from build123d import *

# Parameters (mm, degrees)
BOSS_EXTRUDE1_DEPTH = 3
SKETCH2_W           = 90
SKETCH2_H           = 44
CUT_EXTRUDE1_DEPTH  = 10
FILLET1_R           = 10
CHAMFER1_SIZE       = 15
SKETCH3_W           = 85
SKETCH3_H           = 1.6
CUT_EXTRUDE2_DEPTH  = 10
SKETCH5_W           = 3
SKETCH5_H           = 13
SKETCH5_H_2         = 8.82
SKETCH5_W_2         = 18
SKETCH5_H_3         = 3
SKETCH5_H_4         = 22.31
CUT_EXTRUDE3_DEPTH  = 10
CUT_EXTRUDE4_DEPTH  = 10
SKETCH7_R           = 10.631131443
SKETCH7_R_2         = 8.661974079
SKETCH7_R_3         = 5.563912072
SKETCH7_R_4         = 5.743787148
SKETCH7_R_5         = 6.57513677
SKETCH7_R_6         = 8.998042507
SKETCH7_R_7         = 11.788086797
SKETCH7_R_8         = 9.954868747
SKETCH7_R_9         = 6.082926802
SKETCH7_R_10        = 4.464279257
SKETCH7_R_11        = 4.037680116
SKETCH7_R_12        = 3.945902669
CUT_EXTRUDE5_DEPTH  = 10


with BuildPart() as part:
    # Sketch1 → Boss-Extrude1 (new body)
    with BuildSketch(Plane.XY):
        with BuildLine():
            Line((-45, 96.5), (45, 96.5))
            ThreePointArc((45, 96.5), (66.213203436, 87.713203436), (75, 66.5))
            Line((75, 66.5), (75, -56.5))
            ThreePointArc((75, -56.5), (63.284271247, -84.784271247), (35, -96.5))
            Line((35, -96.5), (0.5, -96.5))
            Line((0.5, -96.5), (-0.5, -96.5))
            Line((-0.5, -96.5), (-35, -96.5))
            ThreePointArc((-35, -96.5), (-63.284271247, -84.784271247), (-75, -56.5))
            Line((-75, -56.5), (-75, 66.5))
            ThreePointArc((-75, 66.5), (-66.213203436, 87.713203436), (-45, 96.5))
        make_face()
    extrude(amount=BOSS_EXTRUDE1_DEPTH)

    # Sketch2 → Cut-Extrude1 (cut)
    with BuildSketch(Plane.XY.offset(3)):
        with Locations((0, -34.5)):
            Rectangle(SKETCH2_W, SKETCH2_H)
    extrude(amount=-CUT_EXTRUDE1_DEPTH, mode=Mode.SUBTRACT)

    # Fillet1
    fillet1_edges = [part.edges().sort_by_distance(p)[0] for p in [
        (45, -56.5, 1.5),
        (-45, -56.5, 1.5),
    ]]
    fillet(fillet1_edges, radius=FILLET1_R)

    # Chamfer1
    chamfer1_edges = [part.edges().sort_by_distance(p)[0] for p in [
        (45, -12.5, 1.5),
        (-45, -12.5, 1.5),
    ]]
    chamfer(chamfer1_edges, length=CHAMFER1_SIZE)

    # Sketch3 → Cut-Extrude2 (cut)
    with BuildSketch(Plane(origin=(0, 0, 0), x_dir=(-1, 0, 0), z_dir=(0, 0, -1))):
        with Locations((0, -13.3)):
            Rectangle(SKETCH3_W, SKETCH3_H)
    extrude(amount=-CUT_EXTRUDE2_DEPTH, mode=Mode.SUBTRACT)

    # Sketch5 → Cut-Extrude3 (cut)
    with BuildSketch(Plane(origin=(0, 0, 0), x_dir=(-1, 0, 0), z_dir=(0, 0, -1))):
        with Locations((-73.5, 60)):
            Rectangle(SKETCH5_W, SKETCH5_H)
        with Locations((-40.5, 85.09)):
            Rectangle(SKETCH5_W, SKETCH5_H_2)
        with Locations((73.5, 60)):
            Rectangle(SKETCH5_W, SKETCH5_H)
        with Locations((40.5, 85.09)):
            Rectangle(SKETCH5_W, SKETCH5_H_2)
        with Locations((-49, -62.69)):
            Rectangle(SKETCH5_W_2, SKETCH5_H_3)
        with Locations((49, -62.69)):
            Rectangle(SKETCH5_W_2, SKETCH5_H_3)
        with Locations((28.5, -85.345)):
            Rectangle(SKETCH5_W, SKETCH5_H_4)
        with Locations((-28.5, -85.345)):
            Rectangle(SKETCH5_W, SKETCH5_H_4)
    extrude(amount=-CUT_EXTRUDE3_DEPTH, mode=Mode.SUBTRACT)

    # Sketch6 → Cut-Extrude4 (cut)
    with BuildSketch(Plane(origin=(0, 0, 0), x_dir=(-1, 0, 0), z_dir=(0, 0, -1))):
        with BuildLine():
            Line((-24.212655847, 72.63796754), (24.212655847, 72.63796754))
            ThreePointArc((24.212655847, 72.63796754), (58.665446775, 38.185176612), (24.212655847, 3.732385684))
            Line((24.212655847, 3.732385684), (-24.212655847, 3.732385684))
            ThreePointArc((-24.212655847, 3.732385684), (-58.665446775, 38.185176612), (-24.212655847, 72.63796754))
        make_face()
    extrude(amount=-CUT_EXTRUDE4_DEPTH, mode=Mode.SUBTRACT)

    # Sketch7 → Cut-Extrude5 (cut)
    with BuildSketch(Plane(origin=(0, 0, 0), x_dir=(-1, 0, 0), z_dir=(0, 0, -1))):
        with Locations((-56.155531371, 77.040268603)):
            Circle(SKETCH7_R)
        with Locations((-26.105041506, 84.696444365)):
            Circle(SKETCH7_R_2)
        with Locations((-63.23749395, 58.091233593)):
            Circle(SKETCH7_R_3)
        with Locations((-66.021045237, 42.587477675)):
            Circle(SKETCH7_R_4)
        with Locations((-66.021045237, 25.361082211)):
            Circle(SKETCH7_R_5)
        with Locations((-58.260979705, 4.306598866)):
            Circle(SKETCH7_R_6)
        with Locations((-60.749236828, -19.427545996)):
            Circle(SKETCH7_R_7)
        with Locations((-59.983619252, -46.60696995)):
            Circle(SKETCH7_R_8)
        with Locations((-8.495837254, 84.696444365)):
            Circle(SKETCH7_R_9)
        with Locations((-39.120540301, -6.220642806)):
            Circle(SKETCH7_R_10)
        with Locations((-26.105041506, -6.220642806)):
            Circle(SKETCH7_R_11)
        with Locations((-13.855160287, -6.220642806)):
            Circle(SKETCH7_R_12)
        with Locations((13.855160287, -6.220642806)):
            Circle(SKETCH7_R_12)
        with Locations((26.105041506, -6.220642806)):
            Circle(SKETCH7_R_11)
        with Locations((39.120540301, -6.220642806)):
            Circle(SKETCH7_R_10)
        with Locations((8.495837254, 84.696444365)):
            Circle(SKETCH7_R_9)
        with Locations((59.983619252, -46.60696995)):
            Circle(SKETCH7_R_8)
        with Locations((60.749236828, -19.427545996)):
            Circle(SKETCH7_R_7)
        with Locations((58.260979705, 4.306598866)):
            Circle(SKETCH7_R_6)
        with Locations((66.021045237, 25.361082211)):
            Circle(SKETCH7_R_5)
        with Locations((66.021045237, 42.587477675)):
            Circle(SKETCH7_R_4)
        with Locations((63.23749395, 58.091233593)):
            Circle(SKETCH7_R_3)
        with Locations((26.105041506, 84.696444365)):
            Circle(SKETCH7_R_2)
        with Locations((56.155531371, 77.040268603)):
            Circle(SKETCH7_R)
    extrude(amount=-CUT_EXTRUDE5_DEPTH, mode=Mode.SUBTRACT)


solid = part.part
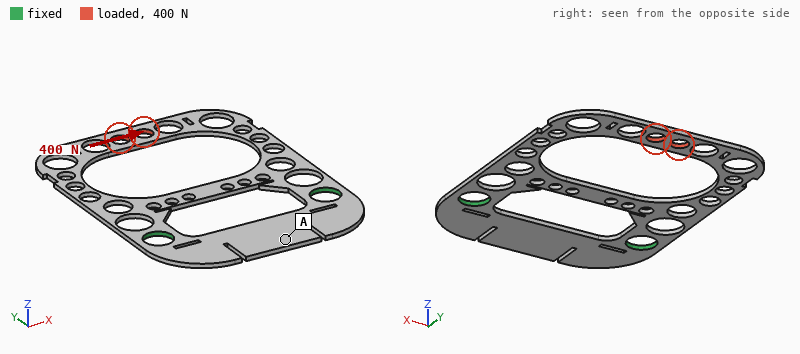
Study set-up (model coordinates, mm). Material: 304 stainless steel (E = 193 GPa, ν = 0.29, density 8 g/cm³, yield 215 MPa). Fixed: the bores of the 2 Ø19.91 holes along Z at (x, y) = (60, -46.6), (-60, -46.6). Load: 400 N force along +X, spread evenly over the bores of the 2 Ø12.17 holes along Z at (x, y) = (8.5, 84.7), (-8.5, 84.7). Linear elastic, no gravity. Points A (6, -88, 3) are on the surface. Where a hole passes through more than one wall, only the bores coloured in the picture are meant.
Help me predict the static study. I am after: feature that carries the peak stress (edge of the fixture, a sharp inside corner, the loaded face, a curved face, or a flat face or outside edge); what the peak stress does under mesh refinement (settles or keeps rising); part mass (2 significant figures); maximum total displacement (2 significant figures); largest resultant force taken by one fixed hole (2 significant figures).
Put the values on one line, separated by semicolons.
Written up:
a sharp inside corner; keeps rising; 290 g; 87 µm; 320 N
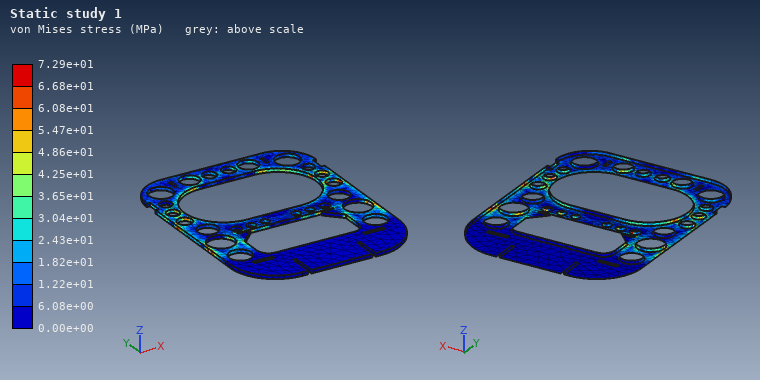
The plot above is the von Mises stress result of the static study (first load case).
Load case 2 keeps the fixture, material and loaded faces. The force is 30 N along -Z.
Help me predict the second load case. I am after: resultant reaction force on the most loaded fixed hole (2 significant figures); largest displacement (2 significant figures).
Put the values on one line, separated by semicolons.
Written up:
15 N; 2.2 mm
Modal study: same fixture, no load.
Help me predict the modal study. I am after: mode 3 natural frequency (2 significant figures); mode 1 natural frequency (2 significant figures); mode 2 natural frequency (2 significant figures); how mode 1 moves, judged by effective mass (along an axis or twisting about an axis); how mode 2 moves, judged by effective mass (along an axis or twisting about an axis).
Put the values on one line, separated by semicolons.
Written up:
510 Hz; 85 Hz; 230 Hz; along Z; twisting about Y
